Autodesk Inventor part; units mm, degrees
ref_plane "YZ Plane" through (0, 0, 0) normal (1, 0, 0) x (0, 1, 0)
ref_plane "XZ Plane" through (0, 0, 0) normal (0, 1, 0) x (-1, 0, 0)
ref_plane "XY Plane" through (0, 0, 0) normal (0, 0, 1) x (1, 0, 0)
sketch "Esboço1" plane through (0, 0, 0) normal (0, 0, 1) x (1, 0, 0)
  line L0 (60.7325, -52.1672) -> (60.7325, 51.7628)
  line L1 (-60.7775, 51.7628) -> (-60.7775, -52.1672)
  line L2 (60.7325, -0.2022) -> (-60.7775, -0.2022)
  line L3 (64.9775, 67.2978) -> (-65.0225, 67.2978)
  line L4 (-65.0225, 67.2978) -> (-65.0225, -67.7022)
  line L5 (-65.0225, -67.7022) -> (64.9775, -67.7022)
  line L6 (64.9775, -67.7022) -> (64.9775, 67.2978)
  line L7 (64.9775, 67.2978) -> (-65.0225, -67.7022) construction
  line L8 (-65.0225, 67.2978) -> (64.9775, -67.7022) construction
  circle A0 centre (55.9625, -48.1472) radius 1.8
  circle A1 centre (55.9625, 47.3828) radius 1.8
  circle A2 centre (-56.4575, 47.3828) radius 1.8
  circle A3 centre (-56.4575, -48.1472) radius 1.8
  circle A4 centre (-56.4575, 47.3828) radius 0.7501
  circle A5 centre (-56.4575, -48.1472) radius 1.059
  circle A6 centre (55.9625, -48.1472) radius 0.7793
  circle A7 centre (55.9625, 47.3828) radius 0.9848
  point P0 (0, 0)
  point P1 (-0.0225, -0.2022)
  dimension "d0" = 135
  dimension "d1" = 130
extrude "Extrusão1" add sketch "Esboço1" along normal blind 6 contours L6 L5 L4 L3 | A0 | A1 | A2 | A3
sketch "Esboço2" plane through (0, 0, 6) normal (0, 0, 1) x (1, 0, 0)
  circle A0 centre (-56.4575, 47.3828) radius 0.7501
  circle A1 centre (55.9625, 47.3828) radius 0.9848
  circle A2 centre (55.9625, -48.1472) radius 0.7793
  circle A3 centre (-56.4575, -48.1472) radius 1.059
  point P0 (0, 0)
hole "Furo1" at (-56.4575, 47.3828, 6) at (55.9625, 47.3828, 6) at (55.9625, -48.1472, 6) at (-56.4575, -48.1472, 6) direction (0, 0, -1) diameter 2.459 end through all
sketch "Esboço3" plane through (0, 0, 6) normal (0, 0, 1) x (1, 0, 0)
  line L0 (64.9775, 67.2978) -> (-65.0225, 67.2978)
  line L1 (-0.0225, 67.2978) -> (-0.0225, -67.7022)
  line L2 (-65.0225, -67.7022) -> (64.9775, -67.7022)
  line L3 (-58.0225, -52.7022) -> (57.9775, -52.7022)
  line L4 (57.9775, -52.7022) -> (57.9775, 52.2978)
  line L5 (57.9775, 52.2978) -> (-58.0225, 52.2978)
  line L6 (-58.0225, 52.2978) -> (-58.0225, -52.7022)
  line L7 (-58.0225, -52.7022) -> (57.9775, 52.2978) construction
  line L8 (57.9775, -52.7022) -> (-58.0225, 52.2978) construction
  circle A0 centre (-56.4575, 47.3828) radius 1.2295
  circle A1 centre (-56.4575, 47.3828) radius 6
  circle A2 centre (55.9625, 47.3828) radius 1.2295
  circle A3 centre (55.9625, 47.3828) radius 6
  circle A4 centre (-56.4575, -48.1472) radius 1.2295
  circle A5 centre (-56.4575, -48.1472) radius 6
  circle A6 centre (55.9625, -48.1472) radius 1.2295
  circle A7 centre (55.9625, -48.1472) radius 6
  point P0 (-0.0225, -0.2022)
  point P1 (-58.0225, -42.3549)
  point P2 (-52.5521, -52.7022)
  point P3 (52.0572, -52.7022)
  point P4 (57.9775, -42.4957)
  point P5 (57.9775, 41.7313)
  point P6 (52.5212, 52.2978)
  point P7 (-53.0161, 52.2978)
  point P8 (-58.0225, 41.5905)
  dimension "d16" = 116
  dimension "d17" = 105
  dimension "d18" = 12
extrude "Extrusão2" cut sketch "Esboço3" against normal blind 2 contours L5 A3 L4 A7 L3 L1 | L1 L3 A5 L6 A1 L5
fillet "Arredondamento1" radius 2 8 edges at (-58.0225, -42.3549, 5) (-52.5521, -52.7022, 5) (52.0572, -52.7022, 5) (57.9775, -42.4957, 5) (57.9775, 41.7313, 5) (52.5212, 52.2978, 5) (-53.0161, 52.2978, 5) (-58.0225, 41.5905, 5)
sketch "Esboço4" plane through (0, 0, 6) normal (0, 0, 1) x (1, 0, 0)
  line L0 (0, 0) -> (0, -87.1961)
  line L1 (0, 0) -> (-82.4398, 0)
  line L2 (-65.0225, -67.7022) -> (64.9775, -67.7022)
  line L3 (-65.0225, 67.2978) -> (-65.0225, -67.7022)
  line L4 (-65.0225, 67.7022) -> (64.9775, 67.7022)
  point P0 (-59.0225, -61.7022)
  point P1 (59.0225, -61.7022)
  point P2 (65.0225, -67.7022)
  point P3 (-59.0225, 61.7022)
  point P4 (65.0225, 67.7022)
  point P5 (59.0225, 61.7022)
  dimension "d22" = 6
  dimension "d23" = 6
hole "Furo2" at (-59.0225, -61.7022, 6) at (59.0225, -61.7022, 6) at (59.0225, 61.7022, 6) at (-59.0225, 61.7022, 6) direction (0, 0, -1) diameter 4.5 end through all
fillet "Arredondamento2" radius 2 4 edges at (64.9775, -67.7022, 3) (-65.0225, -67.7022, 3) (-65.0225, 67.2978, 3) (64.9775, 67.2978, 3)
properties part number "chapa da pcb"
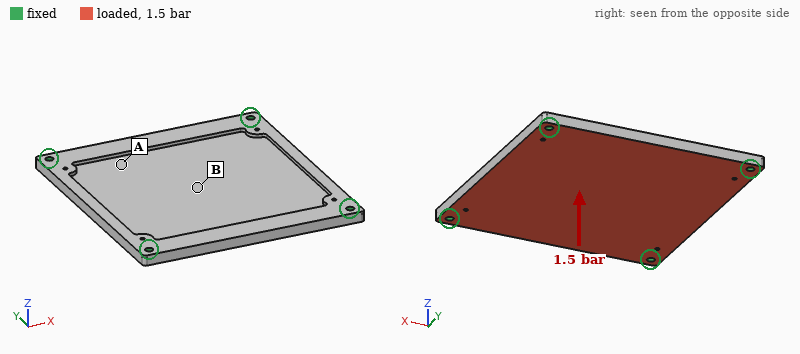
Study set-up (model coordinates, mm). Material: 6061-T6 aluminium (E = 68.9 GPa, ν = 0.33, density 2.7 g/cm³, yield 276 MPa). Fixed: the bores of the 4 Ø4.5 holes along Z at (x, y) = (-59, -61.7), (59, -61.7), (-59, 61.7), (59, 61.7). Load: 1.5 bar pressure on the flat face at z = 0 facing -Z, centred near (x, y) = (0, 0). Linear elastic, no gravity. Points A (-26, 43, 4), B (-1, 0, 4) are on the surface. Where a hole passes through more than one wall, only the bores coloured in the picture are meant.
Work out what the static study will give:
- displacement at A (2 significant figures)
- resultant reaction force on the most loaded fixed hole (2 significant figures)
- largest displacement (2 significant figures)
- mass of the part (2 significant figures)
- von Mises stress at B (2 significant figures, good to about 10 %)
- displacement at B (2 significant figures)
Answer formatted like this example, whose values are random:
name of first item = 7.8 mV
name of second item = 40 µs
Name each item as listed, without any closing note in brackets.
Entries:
displacement at A = 0.19 mm
resultant reaction force on the most loaded fixed hole = 1.0 kN
largest displacement = 0.39 mm
mass of the part = 220 g
von Mises stress at B = 33 MPa
displacement at B = 0.39 mm
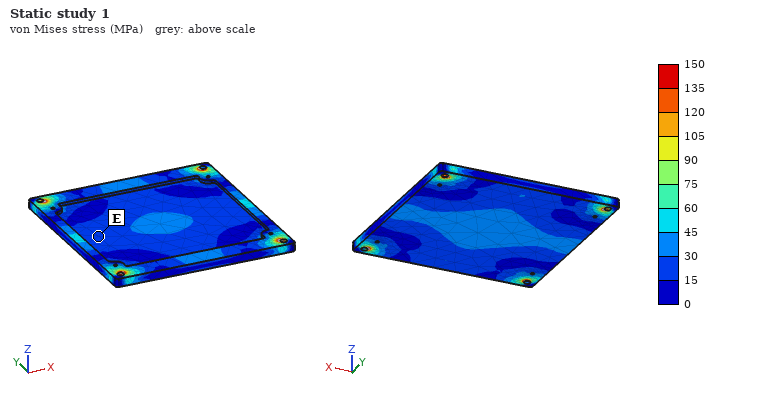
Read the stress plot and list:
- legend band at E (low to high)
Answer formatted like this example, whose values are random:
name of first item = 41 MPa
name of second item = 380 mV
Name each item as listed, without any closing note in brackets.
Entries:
legend band at E = 15 to 30 MPa
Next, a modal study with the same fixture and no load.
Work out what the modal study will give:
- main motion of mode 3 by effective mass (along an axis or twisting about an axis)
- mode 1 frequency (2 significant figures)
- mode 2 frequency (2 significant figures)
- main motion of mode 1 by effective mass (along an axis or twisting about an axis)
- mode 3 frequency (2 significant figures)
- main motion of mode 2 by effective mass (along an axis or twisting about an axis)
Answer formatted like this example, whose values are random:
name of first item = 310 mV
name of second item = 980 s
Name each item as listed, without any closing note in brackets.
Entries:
main motion of mode 3 by effective mass = twisting about X
mode 1 frequency = 1200 Hz
mode 2 frequency = 2000 Hz
main motion of mode 1 by effective mass = along Z
mode 3 frequency = 2100 Hz
main motion of mode 2 by effective mass = twisting about Y
